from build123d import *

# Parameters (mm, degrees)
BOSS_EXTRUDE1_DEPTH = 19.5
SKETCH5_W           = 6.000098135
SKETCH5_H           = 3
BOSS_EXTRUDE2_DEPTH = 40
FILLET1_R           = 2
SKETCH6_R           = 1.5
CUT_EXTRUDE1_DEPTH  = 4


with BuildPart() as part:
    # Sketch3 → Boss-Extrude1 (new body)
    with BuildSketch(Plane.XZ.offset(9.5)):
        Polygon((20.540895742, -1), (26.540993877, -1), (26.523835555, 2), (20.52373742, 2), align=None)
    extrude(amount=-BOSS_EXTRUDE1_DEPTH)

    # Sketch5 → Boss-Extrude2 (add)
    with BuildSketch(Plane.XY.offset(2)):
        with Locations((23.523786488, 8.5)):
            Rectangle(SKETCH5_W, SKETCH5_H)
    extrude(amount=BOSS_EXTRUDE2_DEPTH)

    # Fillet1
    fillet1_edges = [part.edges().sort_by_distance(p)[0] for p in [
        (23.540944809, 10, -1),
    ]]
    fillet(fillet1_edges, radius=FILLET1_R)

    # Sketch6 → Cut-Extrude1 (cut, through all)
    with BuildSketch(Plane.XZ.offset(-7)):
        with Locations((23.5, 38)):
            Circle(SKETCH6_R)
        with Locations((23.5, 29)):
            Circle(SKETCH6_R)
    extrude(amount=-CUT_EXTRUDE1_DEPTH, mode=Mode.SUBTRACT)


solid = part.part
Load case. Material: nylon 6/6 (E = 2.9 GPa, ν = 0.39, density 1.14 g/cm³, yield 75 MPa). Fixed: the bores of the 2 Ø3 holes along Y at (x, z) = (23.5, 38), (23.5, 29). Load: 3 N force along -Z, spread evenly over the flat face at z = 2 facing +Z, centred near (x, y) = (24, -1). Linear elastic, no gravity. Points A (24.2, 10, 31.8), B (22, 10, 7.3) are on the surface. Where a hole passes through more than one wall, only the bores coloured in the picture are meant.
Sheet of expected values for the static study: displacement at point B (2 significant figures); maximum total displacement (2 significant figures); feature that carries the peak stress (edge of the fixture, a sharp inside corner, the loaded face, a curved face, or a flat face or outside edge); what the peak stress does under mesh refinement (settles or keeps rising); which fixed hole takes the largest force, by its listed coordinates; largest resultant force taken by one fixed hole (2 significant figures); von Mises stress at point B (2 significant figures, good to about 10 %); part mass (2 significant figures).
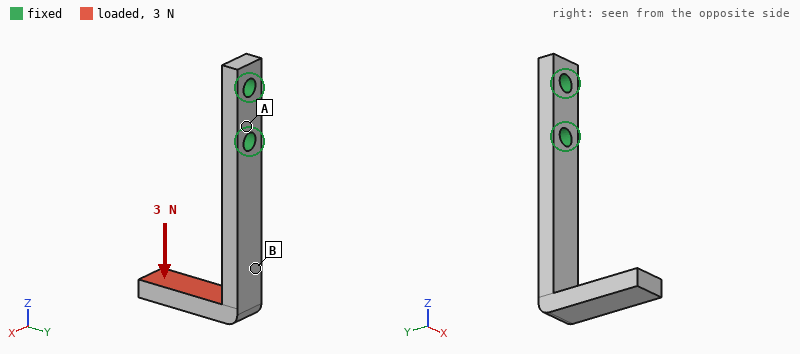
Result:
0.16 mm
0.53 mm
edge of the fixture
keeps rising
(23.5, 29)
2.9 N
3.1 MPa
1.2 g
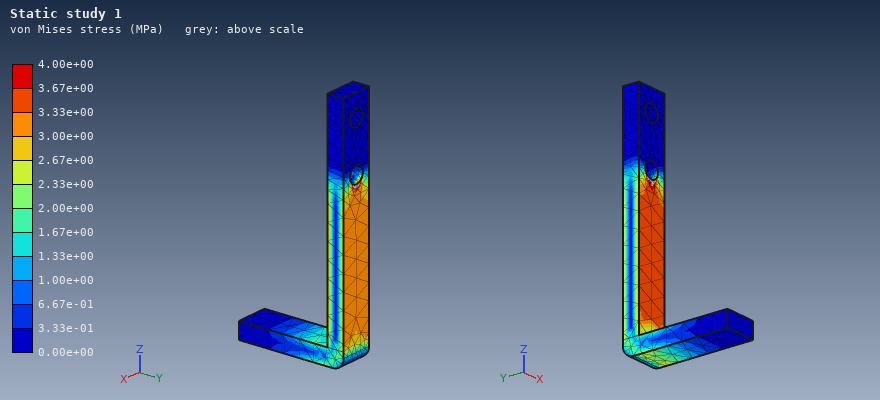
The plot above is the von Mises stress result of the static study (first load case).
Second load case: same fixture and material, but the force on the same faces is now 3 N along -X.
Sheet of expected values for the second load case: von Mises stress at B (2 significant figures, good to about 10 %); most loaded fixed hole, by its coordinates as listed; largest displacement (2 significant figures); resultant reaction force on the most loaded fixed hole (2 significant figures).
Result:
2.7 MPa
(23.5, 29)
0.52 mm
4.8 N
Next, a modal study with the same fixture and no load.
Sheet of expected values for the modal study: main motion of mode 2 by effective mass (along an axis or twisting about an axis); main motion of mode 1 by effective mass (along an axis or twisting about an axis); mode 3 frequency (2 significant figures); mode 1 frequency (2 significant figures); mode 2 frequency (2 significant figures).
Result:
along X
along Y
1600 Hz
480 Hz
730 Hz
